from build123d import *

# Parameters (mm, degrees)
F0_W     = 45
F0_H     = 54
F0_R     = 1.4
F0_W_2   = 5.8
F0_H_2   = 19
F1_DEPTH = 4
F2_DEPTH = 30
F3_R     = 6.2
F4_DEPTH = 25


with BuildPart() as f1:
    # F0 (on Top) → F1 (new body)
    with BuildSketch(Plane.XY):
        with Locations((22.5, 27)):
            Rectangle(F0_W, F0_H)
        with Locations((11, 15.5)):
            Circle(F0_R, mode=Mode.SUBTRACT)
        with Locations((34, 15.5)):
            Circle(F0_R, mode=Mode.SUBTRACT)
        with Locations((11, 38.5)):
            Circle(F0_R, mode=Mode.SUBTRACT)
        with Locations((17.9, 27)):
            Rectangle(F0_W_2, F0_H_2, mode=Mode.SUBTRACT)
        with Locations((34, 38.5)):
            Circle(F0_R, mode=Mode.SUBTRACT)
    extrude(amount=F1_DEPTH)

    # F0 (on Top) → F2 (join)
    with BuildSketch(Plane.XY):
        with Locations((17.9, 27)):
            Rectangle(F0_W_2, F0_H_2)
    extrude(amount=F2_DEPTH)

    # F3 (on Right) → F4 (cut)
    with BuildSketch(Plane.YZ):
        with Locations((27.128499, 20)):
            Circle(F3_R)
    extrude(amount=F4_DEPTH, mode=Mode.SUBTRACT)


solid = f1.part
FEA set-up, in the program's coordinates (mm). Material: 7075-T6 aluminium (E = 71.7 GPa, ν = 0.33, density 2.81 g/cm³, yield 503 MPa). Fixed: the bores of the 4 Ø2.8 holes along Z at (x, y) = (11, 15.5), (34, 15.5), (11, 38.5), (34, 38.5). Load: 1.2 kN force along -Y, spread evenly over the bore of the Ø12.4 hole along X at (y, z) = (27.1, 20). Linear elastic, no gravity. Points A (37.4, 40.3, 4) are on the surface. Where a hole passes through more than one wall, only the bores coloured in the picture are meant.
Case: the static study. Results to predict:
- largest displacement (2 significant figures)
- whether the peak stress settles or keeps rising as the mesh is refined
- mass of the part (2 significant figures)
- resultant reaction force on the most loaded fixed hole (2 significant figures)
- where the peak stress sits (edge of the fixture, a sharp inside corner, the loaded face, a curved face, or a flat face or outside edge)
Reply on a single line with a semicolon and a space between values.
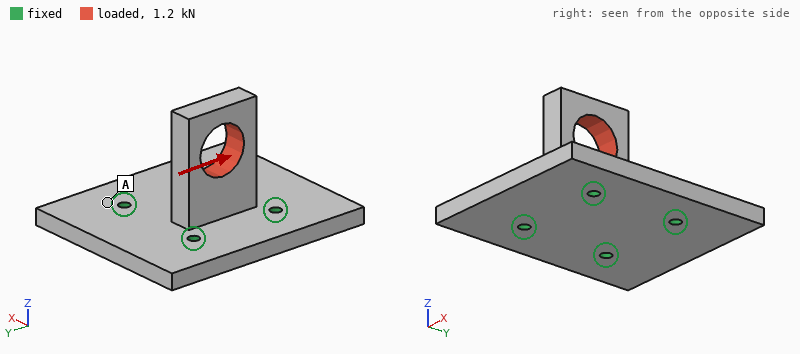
84 µm; keeps rising; 33 g; 900 N; edge of the fixture
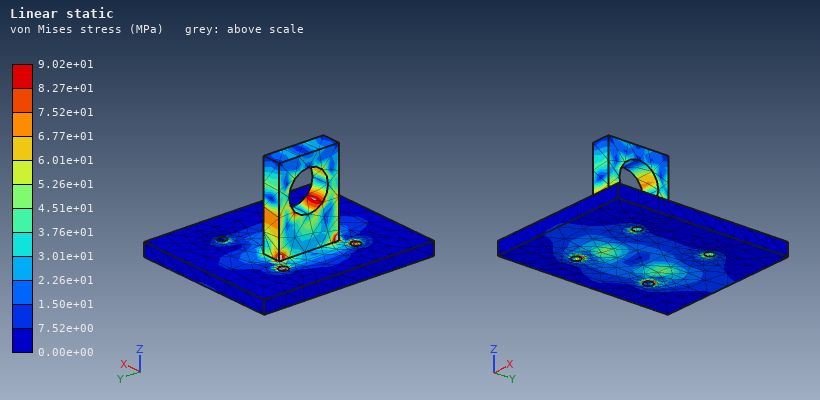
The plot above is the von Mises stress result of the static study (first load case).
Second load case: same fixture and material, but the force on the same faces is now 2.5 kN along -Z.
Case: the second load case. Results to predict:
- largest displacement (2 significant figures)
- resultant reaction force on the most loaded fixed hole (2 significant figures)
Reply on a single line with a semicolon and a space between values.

41 µm; 940 N
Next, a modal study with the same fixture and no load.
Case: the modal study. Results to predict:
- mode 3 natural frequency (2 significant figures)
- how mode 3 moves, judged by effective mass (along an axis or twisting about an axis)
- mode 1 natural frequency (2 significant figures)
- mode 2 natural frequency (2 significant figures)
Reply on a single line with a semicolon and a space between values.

11 kHz; along Z; 5600 Hz; 10 kHz
